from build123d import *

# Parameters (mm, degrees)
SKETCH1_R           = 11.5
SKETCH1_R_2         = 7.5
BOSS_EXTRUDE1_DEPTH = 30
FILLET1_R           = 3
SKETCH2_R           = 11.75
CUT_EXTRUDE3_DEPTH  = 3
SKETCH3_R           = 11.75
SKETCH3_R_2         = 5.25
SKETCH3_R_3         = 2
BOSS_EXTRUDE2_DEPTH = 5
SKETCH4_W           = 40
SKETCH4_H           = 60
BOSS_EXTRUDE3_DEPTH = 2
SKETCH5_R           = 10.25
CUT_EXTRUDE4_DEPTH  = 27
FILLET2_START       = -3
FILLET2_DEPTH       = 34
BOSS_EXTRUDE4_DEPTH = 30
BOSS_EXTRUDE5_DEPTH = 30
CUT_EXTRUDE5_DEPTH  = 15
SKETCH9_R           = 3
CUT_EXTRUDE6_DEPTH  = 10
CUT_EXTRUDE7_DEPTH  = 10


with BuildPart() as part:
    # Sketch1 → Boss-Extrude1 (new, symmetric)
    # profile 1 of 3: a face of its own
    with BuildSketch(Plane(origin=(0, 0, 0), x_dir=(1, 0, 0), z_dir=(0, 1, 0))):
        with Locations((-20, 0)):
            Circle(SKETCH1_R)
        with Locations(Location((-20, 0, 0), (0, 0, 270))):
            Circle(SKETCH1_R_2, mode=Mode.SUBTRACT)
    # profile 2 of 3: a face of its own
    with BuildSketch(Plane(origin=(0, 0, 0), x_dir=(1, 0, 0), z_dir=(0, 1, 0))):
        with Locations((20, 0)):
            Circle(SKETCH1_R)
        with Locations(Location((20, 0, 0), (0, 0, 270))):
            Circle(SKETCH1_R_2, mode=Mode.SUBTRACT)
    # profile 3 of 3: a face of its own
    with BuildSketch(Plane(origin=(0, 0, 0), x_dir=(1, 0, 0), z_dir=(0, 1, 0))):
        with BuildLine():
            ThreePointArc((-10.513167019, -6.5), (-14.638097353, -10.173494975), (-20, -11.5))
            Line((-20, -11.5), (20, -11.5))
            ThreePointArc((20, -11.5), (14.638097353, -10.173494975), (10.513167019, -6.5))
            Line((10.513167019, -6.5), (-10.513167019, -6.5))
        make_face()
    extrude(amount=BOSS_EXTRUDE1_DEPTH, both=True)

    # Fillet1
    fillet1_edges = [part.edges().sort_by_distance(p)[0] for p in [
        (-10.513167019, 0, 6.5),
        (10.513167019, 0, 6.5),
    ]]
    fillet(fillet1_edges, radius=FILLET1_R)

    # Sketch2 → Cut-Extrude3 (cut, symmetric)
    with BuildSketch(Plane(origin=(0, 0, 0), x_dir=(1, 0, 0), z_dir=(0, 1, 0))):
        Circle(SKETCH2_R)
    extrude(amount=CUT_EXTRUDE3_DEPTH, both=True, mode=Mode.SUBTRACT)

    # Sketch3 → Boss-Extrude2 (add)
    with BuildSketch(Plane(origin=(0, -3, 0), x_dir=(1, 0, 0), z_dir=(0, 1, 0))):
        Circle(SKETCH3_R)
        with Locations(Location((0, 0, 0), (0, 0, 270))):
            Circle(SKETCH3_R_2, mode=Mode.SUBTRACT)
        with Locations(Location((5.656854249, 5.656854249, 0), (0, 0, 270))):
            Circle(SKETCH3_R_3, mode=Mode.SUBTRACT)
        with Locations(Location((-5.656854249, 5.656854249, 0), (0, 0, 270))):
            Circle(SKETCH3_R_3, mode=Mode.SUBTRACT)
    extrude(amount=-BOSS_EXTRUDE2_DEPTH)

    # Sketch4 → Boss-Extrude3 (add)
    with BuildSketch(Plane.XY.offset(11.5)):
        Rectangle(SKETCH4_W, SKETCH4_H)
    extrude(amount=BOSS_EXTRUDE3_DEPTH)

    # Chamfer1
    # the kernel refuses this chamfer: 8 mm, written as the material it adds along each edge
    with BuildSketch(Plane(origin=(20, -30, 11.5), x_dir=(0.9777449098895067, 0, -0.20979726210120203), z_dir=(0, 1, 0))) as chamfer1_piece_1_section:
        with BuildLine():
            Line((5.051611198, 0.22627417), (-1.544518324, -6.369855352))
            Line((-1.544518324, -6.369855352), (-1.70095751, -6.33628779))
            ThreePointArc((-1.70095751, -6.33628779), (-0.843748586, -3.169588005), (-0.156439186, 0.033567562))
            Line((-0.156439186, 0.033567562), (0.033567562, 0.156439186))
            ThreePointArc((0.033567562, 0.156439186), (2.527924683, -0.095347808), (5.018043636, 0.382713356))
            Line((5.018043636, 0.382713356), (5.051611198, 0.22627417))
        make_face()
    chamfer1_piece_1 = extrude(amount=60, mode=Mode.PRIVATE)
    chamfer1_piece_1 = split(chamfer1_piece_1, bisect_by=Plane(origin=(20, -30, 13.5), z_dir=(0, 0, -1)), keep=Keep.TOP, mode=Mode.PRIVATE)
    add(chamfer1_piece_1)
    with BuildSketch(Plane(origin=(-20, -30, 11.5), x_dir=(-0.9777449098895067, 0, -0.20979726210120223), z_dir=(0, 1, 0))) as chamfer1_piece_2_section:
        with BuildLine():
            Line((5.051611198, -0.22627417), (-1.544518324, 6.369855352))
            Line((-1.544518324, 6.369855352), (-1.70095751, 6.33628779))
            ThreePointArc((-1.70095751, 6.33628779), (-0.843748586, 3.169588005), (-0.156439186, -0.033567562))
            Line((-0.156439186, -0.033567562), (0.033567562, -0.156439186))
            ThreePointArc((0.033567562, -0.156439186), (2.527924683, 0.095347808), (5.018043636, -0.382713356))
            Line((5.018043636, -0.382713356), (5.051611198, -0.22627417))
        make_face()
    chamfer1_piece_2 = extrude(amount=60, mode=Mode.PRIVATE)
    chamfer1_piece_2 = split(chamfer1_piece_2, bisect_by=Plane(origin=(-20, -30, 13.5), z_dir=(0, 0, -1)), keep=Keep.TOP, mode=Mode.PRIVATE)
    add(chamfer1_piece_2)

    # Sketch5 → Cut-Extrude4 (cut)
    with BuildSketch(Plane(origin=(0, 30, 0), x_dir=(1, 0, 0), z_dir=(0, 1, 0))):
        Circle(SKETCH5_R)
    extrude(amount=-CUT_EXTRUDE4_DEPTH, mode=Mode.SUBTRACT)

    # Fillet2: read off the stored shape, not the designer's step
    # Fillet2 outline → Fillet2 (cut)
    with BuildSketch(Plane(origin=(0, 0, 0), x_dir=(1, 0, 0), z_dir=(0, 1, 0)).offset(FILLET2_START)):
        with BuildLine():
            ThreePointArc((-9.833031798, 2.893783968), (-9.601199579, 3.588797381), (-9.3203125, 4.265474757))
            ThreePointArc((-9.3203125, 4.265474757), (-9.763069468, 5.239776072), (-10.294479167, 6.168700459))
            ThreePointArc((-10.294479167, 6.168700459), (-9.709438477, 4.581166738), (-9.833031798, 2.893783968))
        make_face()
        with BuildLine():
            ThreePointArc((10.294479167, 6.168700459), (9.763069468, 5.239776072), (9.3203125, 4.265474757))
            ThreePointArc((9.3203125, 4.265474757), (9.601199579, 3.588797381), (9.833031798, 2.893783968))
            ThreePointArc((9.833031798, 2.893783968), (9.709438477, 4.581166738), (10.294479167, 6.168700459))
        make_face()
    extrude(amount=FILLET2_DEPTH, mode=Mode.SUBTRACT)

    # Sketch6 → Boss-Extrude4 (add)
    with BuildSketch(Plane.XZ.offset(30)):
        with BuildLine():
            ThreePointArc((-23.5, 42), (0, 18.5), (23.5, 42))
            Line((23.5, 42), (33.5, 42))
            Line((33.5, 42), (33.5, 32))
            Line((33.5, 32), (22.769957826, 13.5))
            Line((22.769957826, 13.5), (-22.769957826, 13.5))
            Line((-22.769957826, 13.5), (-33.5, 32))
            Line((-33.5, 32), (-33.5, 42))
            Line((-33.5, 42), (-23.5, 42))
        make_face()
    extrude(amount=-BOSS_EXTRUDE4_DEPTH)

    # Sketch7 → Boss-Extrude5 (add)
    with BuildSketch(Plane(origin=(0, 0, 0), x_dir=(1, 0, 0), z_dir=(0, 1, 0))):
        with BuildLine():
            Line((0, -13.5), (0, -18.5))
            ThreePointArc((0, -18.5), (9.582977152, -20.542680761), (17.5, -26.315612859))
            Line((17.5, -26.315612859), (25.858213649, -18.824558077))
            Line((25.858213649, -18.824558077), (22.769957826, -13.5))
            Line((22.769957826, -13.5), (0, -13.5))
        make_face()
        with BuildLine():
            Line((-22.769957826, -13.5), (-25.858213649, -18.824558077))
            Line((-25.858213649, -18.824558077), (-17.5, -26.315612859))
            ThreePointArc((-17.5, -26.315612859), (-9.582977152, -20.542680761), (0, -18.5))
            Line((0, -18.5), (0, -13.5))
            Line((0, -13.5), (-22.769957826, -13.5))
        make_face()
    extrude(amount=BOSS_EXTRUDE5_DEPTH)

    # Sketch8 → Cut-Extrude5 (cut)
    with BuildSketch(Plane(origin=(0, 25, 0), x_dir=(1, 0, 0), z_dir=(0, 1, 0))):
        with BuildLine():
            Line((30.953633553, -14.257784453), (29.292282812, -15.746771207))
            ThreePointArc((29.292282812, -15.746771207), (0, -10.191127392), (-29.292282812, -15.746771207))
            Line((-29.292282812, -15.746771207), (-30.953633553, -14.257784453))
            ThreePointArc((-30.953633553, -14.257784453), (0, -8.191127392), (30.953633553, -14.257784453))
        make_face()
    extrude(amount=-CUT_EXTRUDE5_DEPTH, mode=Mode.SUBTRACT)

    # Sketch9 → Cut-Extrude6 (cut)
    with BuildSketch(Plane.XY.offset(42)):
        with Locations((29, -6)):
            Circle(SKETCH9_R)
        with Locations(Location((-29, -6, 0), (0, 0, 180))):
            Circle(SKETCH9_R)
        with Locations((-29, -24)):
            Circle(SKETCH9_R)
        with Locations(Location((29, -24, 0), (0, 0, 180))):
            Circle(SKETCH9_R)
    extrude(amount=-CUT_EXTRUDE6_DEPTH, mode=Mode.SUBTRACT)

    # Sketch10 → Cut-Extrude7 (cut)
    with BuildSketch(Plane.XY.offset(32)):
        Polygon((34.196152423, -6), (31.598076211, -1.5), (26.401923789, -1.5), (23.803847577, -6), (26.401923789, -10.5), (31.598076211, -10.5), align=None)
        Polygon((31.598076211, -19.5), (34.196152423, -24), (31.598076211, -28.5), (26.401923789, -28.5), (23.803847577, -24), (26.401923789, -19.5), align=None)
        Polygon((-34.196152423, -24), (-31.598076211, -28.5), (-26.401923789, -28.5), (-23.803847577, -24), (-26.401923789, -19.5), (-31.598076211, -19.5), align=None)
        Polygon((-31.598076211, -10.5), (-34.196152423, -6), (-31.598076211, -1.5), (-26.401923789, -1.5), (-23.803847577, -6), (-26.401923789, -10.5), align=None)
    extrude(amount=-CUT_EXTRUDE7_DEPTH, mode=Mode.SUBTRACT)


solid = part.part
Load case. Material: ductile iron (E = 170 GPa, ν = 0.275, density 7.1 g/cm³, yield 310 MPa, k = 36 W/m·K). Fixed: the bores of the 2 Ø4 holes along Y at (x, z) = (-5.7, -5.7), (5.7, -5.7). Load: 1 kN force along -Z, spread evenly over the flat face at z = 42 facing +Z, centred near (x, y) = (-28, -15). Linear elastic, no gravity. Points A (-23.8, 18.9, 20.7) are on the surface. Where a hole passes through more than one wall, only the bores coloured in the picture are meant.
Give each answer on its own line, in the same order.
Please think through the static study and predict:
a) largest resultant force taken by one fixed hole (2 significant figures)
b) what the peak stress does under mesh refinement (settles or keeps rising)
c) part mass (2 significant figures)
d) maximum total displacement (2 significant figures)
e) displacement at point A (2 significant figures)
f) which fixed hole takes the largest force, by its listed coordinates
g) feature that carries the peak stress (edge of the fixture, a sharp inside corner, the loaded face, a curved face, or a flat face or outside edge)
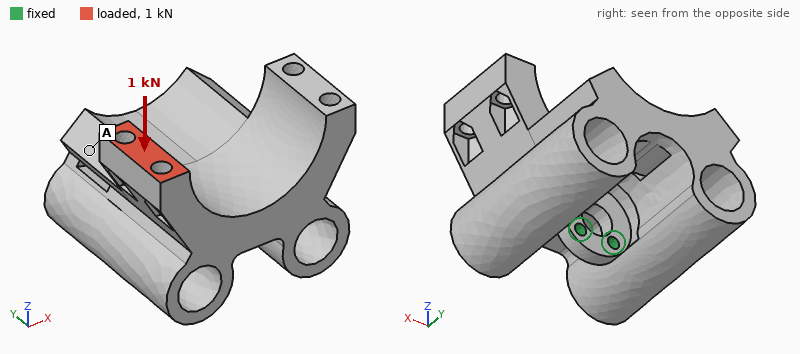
2.2 kN
keeps rising
530 g
96 µm
46 µm
(-5.7, -5.7)
a sharp inside corner
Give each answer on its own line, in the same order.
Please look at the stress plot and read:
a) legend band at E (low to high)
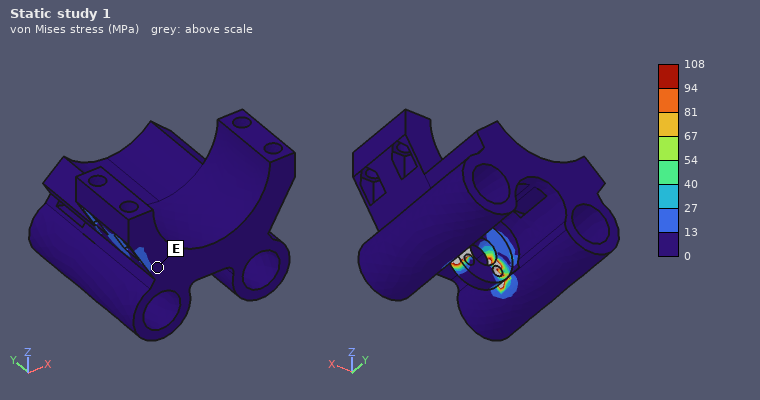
0 to 13 MPa
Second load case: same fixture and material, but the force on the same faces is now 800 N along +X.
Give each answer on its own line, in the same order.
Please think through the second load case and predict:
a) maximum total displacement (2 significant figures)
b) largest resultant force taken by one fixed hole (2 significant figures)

62 µm
2.2 kN
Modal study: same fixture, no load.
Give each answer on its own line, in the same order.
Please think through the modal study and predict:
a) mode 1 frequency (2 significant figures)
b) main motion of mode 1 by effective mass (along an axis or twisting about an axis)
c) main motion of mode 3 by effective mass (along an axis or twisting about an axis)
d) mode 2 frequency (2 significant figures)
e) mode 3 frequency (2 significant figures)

670 Hz
along Y
along X
1600 Hz
1800 Hz
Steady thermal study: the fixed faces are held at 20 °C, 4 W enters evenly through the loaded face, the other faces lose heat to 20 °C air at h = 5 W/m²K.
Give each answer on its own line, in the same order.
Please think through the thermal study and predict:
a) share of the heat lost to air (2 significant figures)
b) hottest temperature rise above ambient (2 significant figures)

26 %
22 K
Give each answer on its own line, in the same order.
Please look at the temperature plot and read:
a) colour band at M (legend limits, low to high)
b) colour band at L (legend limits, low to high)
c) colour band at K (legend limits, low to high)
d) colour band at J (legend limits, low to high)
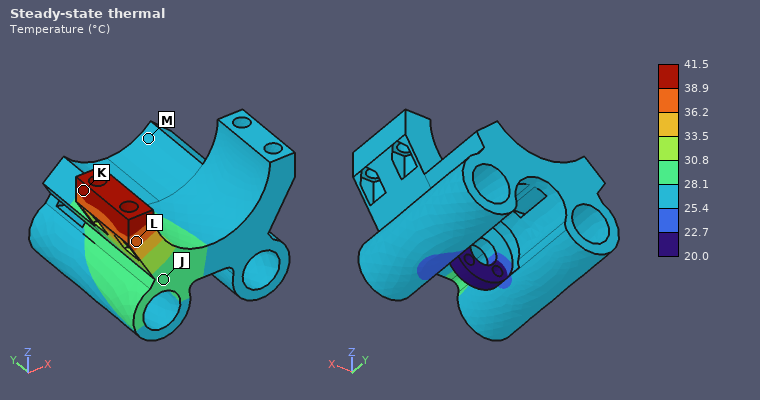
25.4 to 28.1 °C
36.2 to 38.9 °C
38.9 to 41.5 °C
28.1 to 30.8 °C
